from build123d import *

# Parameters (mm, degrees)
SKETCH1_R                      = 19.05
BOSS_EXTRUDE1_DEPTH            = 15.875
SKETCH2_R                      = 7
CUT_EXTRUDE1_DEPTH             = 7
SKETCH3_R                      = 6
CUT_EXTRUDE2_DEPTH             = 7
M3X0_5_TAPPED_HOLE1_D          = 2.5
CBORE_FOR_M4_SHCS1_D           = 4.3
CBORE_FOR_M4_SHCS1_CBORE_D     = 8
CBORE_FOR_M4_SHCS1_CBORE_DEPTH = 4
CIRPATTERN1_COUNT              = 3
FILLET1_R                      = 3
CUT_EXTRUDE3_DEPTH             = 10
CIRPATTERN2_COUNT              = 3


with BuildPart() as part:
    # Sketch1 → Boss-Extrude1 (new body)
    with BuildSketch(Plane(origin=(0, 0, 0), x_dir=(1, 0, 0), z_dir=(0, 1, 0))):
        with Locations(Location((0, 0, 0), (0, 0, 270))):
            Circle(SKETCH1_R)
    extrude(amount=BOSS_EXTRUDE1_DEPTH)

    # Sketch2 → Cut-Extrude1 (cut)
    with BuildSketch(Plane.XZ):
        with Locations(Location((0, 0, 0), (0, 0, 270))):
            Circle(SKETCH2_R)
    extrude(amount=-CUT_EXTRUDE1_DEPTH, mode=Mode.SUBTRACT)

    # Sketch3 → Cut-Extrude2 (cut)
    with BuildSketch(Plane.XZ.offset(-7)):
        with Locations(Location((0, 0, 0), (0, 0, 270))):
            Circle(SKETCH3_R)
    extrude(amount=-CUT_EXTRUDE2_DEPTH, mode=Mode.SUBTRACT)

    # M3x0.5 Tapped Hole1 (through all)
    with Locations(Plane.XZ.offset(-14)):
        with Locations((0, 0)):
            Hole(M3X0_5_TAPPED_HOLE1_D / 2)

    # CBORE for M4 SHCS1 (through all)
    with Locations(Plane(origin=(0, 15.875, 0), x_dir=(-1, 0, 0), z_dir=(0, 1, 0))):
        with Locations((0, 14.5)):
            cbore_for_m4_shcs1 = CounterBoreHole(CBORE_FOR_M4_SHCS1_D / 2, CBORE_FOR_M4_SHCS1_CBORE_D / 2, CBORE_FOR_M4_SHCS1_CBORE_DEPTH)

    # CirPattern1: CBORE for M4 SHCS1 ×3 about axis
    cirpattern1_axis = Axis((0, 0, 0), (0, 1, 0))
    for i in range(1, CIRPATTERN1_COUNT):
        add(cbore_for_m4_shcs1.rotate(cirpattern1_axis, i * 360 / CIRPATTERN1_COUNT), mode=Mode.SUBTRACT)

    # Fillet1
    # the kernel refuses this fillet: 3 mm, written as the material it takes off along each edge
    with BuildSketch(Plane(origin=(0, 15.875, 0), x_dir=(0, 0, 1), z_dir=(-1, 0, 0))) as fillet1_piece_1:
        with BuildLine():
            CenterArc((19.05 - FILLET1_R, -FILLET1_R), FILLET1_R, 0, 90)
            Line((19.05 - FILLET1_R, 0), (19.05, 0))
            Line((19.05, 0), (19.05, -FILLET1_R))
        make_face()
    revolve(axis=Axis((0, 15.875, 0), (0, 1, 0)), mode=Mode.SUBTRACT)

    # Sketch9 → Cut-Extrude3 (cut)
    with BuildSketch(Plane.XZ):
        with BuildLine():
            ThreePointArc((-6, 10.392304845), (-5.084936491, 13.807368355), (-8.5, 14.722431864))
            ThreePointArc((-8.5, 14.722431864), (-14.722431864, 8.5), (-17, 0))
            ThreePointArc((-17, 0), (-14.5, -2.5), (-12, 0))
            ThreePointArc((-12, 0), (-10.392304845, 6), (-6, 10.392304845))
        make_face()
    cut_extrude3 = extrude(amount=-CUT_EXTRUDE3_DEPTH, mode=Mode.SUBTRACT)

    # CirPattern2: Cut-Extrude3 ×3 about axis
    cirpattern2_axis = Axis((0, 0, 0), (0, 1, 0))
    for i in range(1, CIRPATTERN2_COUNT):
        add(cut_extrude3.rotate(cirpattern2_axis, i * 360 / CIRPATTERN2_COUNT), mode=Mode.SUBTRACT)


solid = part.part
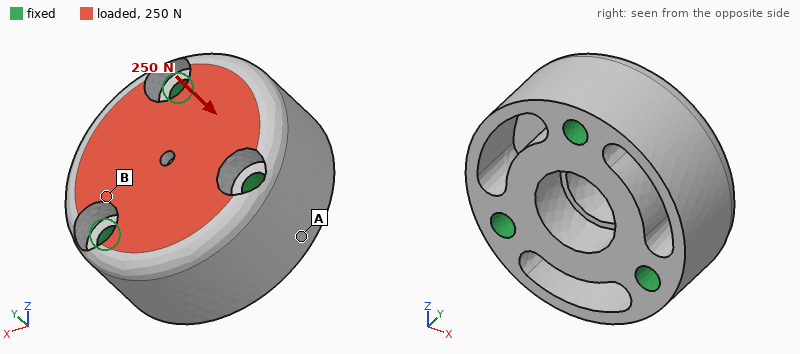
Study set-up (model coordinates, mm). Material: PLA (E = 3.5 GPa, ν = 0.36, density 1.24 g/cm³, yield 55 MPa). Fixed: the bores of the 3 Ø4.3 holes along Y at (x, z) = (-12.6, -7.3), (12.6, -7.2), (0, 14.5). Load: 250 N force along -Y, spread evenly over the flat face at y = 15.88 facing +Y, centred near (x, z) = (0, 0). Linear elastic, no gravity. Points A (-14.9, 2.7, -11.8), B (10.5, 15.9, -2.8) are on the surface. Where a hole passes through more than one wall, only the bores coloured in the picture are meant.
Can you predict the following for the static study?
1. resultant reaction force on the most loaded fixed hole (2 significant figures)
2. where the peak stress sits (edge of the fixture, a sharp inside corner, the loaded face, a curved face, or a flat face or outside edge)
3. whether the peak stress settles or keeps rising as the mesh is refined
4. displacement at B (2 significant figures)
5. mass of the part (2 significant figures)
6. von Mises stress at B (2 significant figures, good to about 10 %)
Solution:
88 N
a sharp inside corner
keeps rising
2.5 µm
15 g
0.54 MPa
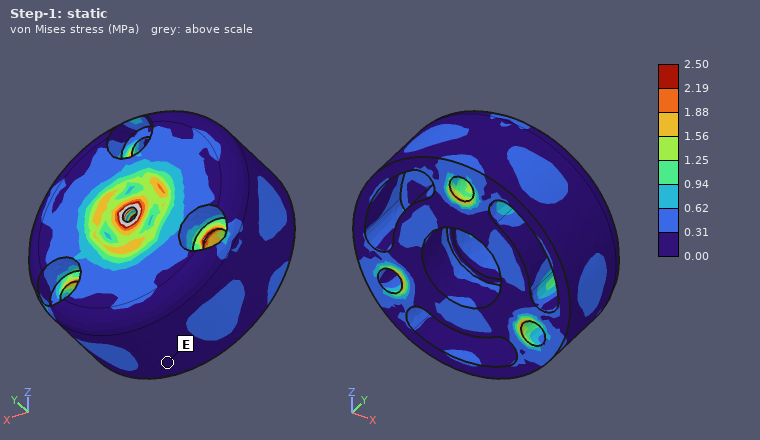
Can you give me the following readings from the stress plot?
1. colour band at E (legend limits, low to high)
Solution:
0.00 to 0.31 MPa
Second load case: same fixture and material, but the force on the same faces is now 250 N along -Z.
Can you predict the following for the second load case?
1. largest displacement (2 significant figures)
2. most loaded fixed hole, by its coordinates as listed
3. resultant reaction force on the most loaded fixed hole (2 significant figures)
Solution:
9.5 µm
(0, 14.5)
110 N
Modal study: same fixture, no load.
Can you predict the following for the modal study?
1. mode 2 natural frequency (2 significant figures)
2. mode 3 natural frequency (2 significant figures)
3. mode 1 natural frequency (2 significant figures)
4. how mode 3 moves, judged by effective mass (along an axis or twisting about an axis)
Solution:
11 kHz
12 kHz
11 kHz
along Y
